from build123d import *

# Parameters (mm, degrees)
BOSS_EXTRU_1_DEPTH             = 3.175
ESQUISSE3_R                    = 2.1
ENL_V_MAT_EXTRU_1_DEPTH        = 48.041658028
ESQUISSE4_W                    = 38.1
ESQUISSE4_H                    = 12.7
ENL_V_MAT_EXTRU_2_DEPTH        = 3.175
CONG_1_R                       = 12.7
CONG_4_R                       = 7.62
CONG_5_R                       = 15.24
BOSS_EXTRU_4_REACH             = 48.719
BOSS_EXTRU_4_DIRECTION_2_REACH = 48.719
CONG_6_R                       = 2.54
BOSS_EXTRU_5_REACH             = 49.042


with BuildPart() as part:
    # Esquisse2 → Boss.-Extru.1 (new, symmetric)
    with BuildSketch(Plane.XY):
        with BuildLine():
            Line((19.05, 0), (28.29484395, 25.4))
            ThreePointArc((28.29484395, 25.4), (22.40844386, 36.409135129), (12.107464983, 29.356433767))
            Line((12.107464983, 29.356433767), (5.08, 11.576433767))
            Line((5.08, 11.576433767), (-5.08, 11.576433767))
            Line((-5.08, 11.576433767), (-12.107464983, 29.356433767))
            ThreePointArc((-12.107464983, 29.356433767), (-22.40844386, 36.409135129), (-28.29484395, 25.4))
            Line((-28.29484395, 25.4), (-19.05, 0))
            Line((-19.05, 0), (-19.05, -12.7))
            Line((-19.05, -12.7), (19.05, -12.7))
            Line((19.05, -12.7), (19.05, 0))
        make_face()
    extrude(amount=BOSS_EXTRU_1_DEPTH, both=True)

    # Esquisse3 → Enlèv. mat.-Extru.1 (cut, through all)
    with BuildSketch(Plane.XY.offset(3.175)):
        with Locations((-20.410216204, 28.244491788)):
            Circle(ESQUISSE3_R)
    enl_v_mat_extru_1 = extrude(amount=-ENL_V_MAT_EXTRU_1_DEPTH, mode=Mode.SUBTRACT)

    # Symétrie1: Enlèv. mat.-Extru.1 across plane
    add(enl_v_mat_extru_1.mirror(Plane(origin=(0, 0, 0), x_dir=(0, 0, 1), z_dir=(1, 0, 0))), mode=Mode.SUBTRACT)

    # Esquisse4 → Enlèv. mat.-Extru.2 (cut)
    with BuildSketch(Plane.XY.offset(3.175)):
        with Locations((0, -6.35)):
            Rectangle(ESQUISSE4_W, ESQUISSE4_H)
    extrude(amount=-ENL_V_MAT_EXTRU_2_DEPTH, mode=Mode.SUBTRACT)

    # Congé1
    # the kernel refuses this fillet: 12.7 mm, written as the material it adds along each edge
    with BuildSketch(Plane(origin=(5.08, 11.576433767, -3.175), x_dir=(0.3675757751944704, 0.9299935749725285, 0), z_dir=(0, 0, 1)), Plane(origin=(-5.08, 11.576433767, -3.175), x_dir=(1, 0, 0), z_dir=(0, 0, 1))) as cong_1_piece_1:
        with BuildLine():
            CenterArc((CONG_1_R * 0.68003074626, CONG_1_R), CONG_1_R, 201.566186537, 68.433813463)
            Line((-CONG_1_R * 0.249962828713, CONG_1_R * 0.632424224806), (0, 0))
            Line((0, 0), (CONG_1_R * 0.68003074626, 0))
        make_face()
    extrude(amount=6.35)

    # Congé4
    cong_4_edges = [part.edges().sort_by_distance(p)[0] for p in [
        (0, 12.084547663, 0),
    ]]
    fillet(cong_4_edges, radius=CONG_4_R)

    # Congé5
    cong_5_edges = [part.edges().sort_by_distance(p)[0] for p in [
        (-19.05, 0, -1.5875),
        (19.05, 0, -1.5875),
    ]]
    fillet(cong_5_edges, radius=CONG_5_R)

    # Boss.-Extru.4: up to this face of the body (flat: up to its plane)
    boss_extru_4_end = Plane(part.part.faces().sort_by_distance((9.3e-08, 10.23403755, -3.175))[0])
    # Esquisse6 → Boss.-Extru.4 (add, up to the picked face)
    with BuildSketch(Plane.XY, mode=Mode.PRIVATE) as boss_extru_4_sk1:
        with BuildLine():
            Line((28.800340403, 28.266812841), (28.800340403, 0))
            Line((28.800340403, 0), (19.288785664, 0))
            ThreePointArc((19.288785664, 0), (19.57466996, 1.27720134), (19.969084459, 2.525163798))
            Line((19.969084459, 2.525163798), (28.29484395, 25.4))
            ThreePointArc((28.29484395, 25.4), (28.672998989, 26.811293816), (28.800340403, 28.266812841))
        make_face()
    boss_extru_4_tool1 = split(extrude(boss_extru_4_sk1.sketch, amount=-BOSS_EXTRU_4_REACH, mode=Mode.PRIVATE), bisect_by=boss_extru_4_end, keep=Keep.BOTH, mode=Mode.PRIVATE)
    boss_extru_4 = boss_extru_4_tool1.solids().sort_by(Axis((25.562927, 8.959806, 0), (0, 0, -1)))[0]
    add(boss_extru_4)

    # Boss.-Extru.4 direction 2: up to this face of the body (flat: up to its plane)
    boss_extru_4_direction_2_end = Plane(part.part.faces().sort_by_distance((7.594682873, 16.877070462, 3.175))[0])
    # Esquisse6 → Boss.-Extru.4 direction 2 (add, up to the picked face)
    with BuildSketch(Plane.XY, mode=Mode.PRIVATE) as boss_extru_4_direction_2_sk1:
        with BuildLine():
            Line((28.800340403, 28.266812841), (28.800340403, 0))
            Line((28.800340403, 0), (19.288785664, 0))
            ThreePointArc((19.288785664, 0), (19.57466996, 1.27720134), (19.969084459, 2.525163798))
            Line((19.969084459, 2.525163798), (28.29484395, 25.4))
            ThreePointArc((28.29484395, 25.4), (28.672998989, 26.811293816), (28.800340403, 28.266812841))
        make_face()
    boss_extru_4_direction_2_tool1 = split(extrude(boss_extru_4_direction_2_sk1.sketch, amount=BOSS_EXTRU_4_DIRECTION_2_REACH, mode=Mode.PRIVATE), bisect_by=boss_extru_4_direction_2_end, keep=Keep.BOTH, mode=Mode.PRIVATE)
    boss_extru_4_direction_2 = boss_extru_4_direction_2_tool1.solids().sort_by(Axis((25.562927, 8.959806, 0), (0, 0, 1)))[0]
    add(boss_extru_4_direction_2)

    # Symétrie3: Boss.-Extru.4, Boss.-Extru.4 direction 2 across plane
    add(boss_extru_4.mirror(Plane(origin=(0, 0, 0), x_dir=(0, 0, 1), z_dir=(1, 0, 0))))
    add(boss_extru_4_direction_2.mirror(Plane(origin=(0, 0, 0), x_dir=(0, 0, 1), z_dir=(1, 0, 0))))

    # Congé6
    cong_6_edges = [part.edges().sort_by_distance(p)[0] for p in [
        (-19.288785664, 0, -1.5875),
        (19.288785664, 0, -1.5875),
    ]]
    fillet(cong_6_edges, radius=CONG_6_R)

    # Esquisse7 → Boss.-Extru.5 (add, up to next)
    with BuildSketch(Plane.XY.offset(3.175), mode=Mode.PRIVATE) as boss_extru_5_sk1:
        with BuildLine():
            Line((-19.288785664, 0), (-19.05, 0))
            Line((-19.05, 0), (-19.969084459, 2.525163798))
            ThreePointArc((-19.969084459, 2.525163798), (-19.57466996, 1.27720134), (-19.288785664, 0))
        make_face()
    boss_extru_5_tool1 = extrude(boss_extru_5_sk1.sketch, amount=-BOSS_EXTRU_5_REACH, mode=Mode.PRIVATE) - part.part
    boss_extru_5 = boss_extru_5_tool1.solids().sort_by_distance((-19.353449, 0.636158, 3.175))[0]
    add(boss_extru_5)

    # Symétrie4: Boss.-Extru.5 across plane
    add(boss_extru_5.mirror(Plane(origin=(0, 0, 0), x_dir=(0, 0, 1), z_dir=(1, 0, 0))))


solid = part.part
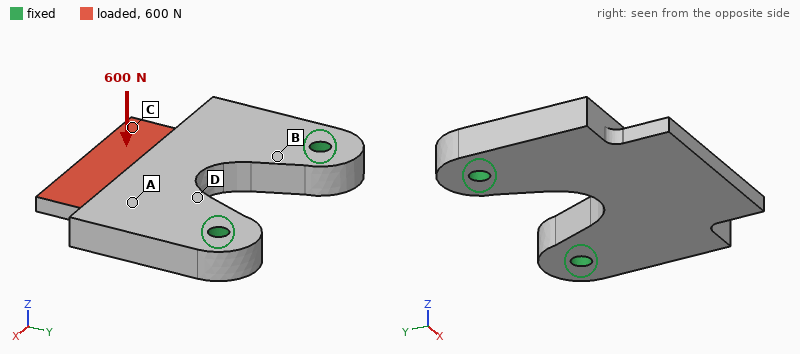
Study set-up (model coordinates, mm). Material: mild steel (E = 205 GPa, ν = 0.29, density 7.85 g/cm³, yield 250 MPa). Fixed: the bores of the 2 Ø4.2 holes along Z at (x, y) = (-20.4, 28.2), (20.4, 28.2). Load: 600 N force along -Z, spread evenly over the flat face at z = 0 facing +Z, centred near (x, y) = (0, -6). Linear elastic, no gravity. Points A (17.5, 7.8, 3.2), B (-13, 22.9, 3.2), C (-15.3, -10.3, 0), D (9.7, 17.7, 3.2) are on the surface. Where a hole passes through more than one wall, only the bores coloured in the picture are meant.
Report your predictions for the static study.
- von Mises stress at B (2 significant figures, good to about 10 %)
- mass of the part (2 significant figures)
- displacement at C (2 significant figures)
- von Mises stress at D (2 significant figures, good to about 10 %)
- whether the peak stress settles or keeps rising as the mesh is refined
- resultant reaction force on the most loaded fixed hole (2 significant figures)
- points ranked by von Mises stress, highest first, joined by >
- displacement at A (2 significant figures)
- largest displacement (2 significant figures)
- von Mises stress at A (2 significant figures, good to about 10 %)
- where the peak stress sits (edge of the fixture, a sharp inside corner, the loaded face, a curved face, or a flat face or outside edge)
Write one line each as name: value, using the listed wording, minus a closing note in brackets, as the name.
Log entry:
von Mises stress at B: 60 MPa
mass of the part: 90 g
displacement at C: 69 µm
von Mises stress at D: 47 MPa
whether the peak stress settles or keeps rising as the mesh is refined: keeps rising
resultant reaction force on the most loaded fixed hole: 300 N
points ranked by von Mises stress, highest first, joined by >: B > D > A > C
displacement at A: 24 µm
largest displacement: 82 µm
von Mises stress at A: 31 MPa
where the peak stress sits: edge of the fixture
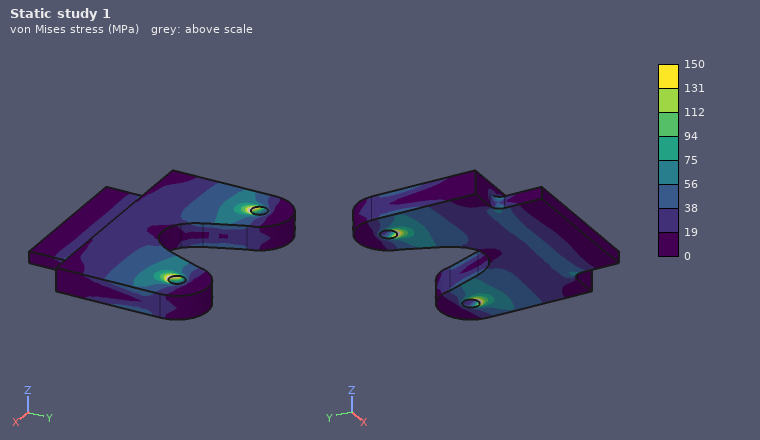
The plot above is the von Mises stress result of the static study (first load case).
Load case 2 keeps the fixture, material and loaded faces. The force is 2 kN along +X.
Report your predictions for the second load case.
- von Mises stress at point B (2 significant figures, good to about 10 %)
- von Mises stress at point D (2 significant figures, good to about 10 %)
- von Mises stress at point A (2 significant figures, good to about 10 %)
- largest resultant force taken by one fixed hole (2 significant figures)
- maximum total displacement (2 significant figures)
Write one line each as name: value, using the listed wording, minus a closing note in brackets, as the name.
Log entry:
von Mises stress at point B: 20 MPa
von Mises stress at point D: 22 MPa
von Mises stress at point A: 7.8 MPa
largest resultant force taken by one fixed hole: 1.8 kN
maximum total displacement: 13 µm
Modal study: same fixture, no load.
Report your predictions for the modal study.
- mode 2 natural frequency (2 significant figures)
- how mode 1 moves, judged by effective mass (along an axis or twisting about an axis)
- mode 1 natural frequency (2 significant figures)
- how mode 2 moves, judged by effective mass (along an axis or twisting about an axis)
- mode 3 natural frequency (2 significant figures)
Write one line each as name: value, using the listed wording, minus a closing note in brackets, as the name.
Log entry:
mode 2 natural frequency: 7200 Hz
how mode 1 moves, judged by effective mass: along Z
mode 1 natural frequency: 3400 Hz
how mode 2 moves, judged by effective mass: twisting about Y
mode 3 natural frequency: 13 kHz
